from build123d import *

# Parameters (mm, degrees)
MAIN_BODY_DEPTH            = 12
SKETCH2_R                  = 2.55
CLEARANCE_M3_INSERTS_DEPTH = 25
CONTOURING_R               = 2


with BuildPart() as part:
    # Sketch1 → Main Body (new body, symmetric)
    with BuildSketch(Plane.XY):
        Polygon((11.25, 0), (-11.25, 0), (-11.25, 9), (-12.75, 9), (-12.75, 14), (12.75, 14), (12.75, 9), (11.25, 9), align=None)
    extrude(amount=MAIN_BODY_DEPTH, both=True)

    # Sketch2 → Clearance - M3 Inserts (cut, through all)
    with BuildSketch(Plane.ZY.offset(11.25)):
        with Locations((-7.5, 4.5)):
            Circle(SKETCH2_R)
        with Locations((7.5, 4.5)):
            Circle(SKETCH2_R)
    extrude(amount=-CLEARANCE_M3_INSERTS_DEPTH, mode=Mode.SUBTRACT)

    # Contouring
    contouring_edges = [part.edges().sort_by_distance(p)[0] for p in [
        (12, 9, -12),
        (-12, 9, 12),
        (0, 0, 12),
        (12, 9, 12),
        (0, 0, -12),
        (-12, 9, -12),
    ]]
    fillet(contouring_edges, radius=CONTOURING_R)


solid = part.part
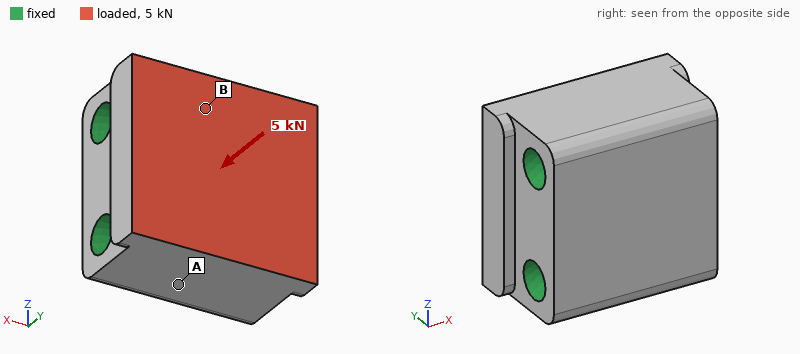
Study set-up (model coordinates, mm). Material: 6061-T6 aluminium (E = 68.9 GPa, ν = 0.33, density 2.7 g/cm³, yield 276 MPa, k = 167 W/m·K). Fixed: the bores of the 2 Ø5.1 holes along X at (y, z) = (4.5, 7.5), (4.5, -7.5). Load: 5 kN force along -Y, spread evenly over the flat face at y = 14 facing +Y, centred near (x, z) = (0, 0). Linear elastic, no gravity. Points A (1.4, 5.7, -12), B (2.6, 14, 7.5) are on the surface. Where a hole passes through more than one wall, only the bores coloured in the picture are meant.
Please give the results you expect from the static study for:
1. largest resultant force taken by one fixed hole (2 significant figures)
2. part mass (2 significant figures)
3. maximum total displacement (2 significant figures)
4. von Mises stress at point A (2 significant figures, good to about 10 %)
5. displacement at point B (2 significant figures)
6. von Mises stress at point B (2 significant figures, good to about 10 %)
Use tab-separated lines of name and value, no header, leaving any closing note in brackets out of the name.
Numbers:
largest resultant force taken by one fixed hole	2.5 kN
part mass	19 g
maximum total displacement	2.1 µm
von Mises stress at point A	4.5 MPa
displacement at point B	0.94 µm
von Mises stress at point B	9.8 MPa
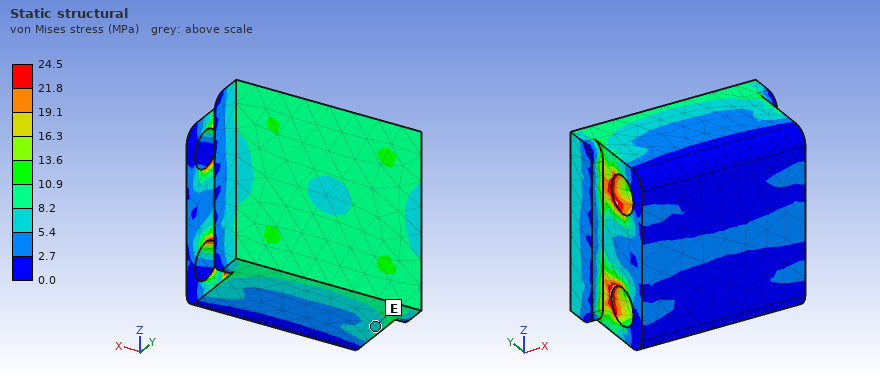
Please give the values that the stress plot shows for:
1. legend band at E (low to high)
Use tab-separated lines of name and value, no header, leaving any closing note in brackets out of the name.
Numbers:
legend band at E	5.4 to 8.2 MPa
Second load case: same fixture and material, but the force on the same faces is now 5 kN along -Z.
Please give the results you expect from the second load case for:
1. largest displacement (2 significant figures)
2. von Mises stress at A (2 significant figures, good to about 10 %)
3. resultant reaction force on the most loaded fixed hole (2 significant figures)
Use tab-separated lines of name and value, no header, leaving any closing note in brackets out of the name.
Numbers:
largest displacement	5.7 µm
von Mises stress at A	16 MPa
resultant reaction force on the most loaded fixed hole	3.3 kN
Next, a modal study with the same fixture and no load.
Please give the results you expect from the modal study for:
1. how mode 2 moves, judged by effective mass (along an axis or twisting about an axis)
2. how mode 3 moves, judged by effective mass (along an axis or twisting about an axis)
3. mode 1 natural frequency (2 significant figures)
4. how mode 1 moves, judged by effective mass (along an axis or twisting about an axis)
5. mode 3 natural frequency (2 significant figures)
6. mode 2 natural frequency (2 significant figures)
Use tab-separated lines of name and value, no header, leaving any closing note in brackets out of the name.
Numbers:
how mode 2 moves, judged by effective mass	along Z
how mode 3 moves, judged by effective mass	twisting about Y
mode 1 natural frequency	71 kHz
how mode 1 moves, judged by effective mass	along X
mode 3 natural frequency	82 kHz
mode 2 natural frequency	78 kHz
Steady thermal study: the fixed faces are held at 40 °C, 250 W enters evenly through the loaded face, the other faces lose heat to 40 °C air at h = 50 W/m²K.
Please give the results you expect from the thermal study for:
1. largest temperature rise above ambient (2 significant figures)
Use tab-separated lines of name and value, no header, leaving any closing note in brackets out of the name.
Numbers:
largest temperature rise above ambient	24 K
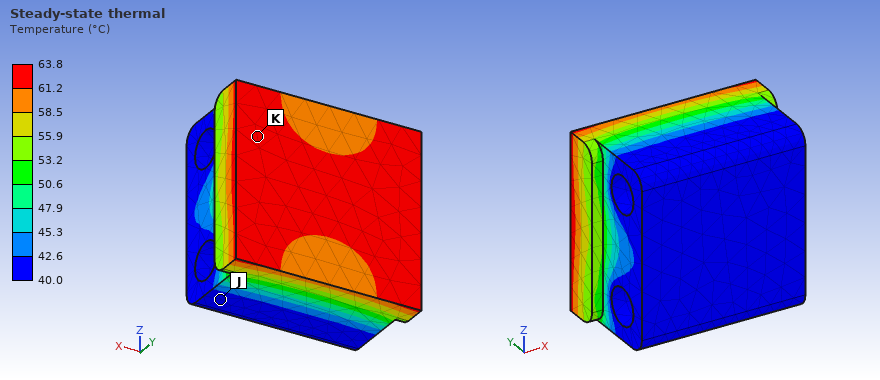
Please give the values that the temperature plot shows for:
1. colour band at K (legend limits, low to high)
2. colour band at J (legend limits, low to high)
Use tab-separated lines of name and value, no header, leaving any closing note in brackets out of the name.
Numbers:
colour band at K	61.2 to 63.8 °C
colour band at J	40.0 to 42.6 °C
